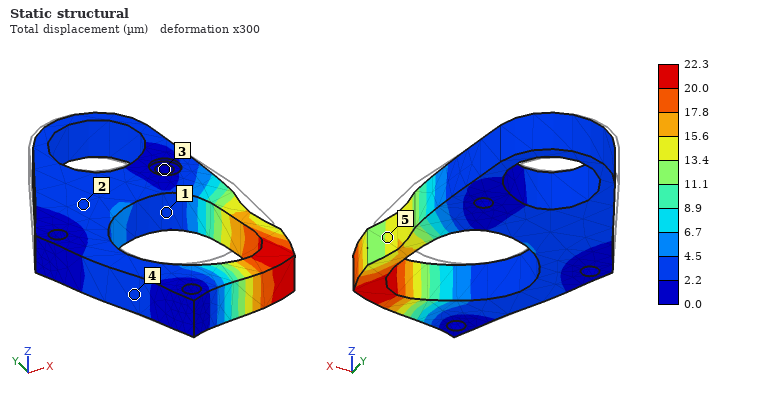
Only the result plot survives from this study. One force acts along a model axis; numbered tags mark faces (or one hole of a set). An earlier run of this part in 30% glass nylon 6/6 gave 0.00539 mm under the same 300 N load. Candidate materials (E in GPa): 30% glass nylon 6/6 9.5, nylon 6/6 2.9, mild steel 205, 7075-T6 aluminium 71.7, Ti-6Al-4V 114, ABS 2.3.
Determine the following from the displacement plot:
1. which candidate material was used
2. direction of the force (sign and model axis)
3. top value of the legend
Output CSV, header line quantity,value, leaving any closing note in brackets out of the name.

quantity,value
which candidate material was used,ABS
direction of the force,-Y
top value of the legend,22.3 µm
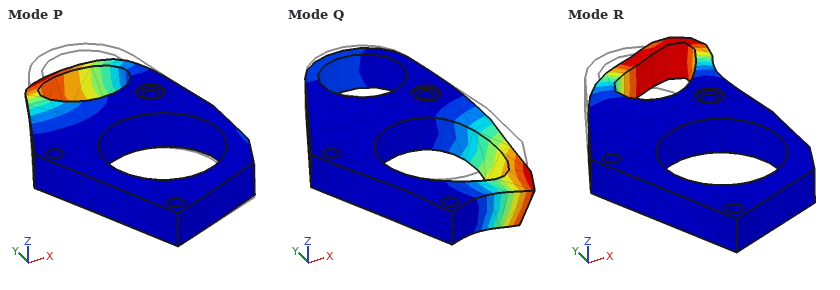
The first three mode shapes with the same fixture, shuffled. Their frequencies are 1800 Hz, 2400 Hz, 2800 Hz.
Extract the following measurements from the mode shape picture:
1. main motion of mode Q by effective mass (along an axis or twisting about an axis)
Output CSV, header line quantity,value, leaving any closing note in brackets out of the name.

quantity,value
main motion of mode Q by effective mass,along Z
